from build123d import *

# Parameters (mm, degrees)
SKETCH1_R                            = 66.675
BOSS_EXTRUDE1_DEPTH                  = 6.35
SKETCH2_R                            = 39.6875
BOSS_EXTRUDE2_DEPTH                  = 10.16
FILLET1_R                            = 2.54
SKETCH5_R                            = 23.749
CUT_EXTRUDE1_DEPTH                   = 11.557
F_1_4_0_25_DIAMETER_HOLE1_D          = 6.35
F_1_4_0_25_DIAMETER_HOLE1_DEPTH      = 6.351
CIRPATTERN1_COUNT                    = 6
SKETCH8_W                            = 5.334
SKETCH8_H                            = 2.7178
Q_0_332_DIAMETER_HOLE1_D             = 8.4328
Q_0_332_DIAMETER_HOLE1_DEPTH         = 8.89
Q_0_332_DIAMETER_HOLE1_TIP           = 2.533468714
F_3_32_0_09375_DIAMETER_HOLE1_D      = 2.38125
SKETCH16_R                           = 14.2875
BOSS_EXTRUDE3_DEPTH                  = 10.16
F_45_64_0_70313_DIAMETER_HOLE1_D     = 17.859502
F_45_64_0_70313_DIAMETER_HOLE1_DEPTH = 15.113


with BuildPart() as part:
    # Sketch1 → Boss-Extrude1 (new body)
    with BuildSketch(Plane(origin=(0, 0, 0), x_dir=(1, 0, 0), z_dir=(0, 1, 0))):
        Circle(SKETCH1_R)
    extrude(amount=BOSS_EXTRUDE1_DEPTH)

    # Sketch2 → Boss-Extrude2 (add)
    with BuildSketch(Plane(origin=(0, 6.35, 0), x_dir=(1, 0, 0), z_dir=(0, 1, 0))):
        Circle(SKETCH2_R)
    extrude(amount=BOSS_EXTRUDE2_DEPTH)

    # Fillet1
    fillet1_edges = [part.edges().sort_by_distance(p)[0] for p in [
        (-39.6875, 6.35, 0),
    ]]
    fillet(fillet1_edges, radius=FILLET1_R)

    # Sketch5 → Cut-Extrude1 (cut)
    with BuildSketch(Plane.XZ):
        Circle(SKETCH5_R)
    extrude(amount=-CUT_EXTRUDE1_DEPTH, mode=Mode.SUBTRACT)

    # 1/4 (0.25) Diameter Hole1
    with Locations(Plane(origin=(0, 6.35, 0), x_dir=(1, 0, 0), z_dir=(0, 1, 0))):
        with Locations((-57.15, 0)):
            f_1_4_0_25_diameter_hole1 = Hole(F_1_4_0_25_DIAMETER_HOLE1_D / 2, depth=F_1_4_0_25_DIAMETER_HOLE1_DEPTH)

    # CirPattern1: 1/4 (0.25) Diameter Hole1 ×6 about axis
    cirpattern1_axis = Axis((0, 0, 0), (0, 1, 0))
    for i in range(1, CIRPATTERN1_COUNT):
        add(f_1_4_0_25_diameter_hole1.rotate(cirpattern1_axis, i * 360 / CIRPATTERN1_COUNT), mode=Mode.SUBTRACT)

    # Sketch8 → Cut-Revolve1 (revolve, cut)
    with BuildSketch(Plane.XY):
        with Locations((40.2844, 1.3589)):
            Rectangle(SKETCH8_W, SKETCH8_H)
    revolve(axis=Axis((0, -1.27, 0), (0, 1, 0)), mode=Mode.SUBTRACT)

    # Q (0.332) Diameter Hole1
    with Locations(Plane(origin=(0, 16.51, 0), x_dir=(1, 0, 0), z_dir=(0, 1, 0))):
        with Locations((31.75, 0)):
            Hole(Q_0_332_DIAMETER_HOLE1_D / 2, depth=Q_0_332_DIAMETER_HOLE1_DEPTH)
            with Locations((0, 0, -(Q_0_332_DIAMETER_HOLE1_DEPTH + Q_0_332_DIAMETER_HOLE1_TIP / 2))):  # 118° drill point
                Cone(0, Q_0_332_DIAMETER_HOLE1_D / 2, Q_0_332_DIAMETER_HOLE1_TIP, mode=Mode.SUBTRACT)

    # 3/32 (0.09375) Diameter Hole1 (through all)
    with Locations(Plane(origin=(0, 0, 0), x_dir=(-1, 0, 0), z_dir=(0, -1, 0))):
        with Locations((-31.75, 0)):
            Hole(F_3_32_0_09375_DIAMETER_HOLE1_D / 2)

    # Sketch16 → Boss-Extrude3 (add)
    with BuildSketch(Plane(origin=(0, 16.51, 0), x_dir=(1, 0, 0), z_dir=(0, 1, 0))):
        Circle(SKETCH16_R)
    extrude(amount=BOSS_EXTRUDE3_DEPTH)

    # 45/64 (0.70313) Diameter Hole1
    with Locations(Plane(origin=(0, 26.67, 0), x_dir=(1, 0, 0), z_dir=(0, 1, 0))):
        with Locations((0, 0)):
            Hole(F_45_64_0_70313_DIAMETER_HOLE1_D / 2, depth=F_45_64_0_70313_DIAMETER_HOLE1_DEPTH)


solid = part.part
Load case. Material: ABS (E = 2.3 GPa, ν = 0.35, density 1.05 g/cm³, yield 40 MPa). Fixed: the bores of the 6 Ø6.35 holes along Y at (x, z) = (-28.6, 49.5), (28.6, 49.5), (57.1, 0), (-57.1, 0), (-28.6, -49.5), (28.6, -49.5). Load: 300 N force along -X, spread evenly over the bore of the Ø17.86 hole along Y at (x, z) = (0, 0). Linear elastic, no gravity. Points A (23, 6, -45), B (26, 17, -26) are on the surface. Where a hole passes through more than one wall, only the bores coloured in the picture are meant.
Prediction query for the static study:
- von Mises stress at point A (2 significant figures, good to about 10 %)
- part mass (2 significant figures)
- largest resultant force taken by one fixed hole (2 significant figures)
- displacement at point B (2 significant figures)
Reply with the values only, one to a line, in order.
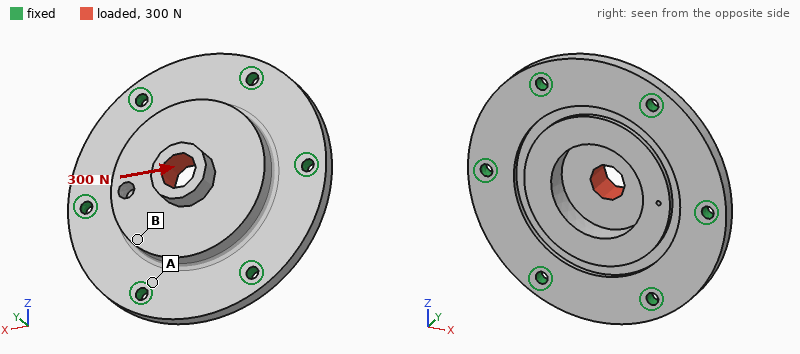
0.44 MPa
120 g
83 N
14 µm
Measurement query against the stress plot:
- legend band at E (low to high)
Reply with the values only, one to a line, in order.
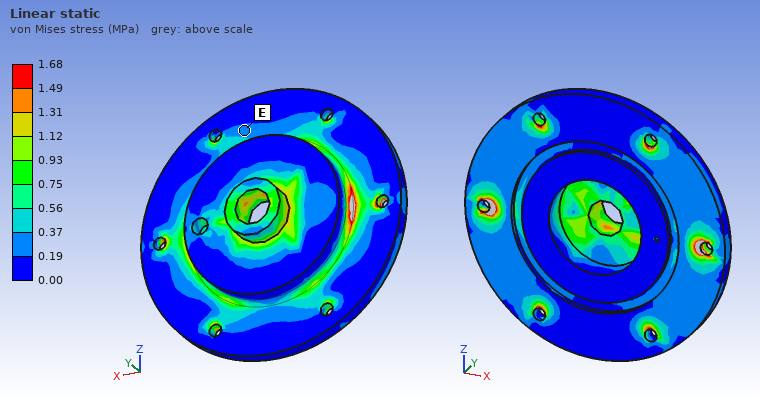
0.19 to 0.37 MPa
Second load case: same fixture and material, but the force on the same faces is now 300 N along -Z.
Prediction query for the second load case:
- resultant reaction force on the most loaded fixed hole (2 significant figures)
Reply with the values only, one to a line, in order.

73 N
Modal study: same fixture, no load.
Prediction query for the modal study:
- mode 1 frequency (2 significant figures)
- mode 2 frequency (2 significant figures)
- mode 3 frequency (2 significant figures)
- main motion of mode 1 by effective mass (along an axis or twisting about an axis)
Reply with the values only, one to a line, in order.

1600 Hz
2200 Hz
2200 Hz
along Y
